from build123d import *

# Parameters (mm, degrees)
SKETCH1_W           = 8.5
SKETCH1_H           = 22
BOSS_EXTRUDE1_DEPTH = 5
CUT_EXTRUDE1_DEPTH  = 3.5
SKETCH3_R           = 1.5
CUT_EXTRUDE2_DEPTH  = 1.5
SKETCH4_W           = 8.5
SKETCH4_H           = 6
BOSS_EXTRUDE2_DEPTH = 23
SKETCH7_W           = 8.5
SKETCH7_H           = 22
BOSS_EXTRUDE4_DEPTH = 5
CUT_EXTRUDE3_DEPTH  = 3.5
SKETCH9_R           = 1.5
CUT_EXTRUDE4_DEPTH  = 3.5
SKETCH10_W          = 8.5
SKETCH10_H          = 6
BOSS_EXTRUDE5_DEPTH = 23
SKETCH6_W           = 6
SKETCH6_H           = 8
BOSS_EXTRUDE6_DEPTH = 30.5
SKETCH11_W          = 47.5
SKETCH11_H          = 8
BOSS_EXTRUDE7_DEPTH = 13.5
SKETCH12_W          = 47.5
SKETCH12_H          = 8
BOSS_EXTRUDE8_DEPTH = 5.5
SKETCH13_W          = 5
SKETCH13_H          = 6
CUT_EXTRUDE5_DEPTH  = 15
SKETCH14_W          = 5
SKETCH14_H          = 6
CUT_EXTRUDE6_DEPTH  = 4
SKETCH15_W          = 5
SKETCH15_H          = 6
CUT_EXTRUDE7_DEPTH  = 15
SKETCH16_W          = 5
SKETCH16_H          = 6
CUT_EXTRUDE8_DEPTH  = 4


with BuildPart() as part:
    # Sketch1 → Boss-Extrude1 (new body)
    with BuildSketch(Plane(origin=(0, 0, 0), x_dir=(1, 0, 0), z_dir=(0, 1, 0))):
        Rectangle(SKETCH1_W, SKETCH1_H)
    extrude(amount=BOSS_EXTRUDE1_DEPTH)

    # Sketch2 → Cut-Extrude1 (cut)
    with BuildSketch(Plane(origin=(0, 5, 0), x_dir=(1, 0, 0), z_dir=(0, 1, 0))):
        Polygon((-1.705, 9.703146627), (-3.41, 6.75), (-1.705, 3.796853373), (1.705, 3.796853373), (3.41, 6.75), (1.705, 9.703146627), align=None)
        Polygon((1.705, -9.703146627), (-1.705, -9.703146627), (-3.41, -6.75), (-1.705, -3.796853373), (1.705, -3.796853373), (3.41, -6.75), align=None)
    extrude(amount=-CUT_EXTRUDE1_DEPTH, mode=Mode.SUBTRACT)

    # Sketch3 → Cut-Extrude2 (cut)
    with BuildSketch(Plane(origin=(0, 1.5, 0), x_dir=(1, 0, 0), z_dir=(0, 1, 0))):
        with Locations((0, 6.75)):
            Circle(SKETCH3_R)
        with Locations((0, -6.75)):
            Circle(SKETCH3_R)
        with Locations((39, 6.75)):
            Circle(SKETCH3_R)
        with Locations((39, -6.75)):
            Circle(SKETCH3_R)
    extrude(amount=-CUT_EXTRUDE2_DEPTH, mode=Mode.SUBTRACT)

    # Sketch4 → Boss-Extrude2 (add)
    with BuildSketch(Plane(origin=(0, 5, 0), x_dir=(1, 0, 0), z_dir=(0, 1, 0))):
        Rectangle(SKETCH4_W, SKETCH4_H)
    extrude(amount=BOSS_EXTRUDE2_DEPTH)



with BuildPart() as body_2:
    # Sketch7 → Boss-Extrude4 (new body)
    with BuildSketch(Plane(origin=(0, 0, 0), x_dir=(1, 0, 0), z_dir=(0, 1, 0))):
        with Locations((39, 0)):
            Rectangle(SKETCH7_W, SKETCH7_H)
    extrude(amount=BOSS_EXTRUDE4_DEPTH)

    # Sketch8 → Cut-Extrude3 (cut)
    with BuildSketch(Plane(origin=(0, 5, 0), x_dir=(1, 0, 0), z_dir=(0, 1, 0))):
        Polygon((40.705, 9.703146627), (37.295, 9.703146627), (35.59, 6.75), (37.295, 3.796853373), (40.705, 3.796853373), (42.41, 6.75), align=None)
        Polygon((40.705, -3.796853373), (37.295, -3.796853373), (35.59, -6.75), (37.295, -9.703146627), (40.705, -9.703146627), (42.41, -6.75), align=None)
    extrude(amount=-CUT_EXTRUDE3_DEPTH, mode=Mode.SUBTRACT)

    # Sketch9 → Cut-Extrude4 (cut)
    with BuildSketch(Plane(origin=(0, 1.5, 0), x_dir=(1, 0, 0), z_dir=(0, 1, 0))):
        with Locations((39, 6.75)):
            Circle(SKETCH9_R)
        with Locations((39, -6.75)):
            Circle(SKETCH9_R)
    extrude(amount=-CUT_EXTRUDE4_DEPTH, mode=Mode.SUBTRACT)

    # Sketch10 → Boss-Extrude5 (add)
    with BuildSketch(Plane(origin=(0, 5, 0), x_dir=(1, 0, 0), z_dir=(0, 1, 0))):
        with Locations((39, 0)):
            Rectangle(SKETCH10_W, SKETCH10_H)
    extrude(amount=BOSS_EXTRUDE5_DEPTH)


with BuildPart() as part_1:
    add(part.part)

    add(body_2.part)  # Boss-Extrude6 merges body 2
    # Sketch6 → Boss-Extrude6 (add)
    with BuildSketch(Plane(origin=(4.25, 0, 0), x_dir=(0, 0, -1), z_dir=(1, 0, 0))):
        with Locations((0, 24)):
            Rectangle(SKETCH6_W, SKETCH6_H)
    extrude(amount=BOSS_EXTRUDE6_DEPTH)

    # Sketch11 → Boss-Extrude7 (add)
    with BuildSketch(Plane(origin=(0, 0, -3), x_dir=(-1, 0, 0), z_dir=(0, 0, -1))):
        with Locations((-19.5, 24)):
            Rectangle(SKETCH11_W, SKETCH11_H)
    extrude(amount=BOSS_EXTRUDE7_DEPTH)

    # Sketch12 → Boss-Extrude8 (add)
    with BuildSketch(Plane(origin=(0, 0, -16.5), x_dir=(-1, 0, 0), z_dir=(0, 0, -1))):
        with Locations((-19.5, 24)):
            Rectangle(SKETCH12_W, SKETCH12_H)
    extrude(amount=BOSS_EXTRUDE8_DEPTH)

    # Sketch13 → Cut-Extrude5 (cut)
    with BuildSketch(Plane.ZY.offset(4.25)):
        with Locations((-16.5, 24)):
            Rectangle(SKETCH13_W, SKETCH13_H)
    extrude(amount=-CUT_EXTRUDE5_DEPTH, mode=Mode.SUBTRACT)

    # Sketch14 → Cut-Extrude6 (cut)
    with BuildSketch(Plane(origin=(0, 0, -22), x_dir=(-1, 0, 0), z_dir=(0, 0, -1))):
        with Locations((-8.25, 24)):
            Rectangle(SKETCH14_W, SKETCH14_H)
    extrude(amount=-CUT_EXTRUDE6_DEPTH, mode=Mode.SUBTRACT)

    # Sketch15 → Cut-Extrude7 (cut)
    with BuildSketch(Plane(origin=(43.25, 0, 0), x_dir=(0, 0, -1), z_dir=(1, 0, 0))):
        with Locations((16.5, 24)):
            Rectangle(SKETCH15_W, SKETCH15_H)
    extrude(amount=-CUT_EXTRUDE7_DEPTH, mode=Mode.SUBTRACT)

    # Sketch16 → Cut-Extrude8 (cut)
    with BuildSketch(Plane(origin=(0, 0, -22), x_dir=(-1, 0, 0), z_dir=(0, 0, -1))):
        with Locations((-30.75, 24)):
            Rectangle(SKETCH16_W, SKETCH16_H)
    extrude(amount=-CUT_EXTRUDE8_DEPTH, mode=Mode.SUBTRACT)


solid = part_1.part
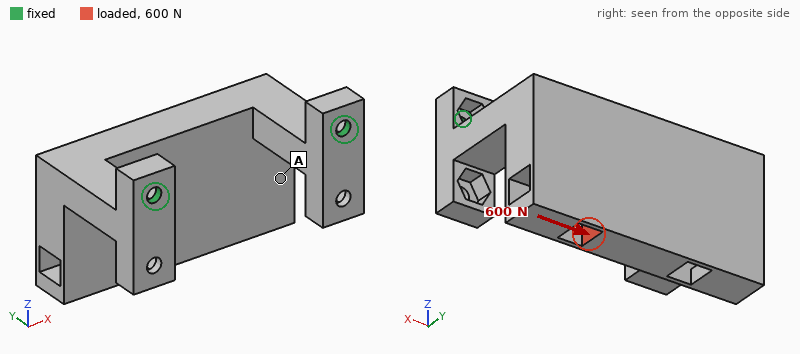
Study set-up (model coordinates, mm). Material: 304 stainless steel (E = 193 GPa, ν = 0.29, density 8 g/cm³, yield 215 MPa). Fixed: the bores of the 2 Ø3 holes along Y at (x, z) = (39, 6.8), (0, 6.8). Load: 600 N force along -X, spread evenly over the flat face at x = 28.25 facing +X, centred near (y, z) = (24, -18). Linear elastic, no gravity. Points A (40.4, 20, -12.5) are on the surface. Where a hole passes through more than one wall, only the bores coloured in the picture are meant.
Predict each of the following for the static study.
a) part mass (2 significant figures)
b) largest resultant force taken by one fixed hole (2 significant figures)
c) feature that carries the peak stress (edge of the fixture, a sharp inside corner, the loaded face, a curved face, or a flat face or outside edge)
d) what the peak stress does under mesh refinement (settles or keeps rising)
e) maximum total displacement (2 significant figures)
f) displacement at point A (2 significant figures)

91 g
500 N
edge of the fixture
keeps rising
51 µm
41 µm
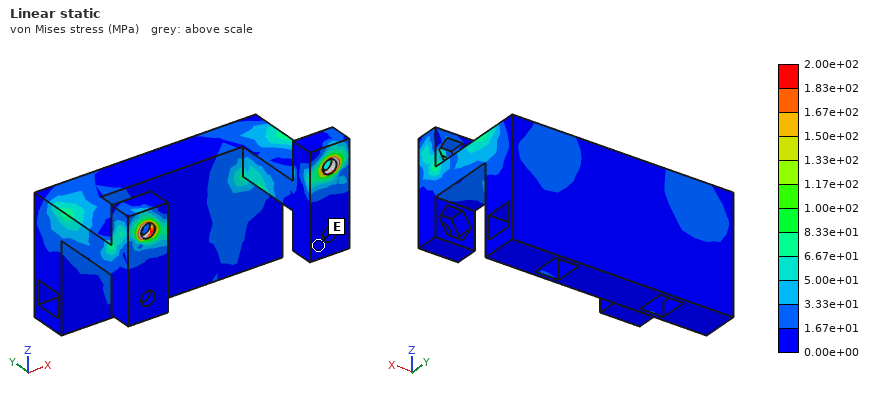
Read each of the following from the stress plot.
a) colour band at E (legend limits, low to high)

0.00e+00 to 1.67e+01 MPa
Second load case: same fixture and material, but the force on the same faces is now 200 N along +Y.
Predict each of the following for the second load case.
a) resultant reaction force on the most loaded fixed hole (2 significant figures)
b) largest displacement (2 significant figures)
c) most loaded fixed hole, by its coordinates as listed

140 N
0.15 mm
(39, 6.8)
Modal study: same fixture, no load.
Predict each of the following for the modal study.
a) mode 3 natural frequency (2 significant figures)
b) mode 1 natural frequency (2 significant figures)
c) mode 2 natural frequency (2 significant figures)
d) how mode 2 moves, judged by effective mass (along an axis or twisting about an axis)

3200 Hz
770 Hz
2700 Hz
along X
